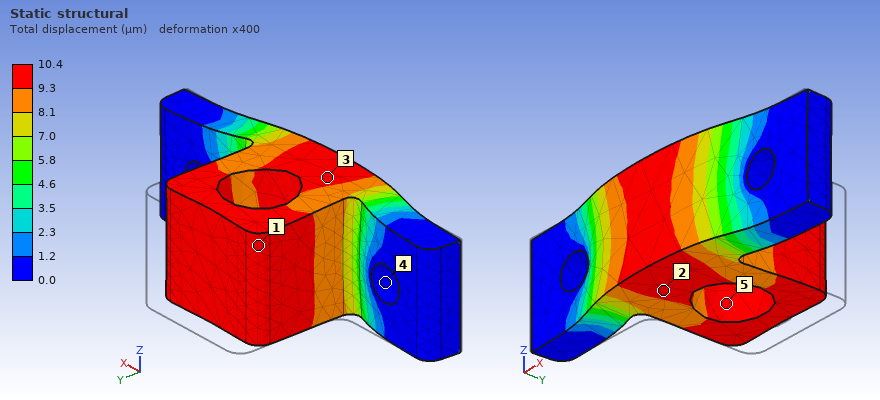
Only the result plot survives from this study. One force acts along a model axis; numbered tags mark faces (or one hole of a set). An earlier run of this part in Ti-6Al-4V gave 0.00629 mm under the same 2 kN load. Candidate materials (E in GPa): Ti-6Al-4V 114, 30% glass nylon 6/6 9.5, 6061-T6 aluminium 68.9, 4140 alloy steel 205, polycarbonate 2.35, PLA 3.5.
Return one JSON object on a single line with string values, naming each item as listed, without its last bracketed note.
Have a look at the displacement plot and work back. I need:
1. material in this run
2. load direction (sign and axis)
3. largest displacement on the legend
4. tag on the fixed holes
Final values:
{"material in this run": "6061-T6 aluminium", "load direction": "-Y", "largest displacement on the legend": "10.4 µm", "tag on the fixed holes": "4"}
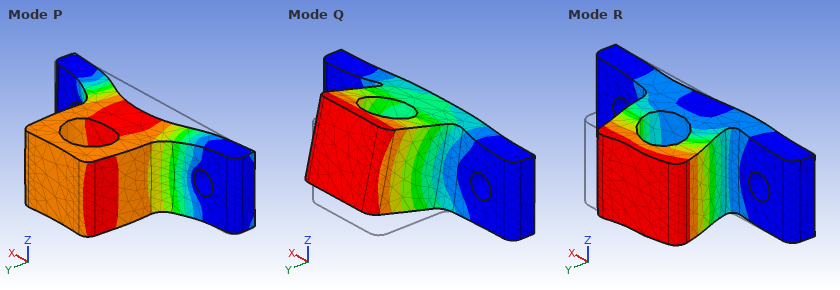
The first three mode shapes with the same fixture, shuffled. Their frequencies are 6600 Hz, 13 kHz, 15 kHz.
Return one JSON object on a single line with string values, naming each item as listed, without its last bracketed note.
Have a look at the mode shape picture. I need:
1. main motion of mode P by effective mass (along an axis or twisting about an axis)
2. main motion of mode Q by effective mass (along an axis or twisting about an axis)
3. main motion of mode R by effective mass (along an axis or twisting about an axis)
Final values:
{"main motion of mode P by effective mass": "along Y", "main motion of mode Q by effective mass": "along Z", "main motion of mode R by effective mass": "along X"}
